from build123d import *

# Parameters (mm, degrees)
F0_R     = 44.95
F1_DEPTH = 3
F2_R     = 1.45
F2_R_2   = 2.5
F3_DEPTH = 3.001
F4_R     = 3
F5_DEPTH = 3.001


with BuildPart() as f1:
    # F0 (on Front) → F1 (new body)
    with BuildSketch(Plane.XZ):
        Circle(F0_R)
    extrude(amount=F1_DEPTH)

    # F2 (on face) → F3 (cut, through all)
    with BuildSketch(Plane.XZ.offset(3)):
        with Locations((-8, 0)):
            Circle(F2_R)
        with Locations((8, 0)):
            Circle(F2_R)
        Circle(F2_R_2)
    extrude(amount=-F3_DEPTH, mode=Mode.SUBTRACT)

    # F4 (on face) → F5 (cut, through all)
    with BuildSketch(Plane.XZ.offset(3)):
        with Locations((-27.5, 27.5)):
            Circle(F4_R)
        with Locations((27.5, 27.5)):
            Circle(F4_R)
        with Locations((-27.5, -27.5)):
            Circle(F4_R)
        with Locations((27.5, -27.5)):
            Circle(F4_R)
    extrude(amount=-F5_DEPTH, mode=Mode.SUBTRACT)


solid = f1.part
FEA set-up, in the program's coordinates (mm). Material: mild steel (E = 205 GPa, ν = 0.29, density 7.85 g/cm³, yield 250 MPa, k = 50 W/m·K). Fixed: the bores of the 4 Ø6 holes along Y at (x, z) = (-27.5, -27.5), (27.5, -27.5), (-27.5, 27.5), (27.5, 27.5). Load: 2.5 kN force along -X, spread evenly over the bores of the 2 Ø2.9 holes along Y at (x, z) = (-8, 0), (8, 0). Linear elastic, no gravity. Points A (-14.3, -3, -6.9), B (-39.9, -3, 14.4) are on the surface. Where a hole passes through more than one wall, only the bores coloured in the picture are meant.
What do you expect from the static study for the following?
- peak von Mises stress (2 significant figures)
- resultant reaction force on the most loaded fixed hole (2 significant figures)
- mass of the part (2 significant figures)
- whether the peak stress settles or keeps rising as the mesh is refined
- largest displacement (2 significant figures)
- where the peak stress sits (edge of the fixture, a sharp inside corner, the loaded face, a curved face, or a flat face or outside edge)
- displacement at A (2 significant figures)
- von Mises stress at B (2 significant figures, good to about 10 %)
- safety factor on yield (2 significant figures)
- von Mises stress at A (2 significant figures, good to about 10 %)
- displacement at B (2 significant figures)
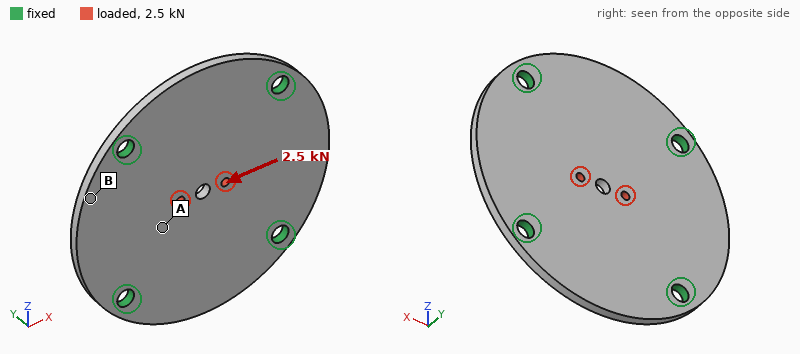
82 MPa
650 N
150 g
settles
3.4 µm
the loaded face
1.9 µm
6.2 MPa
3.0
14 MPa
1.1 µm
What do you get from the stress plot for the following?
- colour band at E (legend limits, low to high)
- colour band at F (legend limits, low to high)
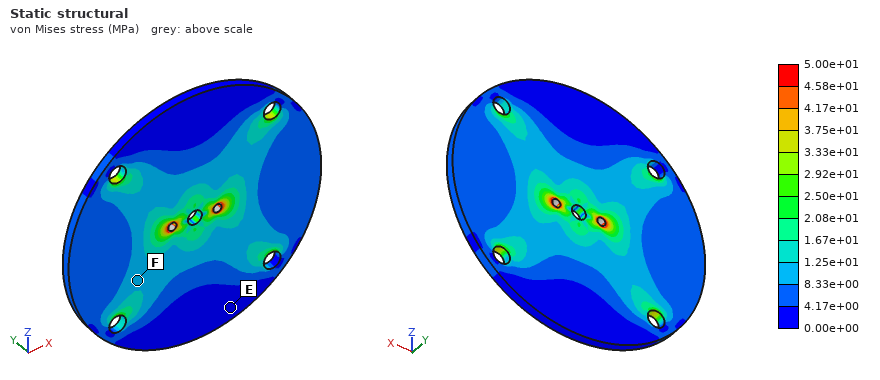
0.00e+00 to 4.17e+00 MPa
8.33e+00 to 1.25e+01 MPa
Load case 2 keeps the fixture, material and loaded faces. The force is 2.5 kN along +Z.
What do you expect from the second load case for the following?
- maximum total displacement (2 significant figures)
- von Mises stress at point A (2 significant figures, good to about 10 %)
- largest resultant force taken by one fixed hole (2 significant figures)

2.9 µm
14 MPa
650 N
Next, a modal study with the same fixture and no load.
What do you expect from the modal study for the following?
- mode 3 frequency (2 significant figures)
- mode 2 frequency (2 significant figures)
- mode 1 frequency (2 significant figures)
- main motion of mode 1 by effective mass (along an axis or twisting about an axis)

4900 Hz
4700 Hz
4000 Hz
along Y
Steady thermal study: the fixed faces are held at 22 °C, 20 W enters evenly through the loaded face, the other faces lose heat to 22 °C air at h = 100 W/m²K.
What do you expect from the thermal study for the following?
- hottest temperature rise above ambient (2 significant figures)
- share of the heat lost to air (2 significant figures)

42 K
54 %
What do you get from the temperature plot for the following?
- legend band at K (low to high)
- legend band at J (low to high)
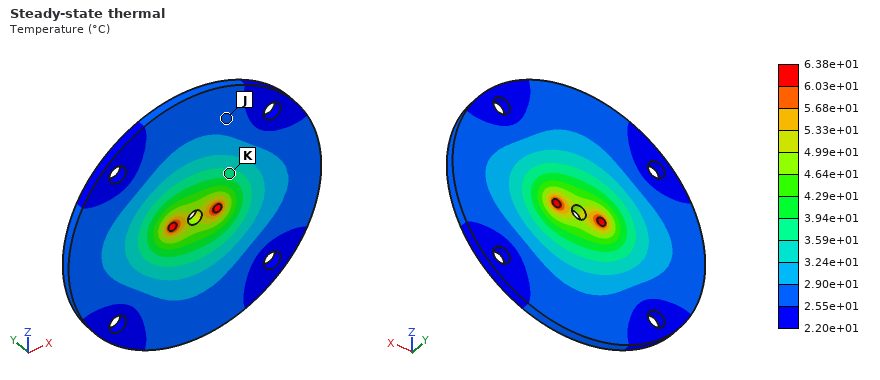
3.59e+01 to 3.94e+01 °C
2.55e+01 to 2.90e+01 °C
